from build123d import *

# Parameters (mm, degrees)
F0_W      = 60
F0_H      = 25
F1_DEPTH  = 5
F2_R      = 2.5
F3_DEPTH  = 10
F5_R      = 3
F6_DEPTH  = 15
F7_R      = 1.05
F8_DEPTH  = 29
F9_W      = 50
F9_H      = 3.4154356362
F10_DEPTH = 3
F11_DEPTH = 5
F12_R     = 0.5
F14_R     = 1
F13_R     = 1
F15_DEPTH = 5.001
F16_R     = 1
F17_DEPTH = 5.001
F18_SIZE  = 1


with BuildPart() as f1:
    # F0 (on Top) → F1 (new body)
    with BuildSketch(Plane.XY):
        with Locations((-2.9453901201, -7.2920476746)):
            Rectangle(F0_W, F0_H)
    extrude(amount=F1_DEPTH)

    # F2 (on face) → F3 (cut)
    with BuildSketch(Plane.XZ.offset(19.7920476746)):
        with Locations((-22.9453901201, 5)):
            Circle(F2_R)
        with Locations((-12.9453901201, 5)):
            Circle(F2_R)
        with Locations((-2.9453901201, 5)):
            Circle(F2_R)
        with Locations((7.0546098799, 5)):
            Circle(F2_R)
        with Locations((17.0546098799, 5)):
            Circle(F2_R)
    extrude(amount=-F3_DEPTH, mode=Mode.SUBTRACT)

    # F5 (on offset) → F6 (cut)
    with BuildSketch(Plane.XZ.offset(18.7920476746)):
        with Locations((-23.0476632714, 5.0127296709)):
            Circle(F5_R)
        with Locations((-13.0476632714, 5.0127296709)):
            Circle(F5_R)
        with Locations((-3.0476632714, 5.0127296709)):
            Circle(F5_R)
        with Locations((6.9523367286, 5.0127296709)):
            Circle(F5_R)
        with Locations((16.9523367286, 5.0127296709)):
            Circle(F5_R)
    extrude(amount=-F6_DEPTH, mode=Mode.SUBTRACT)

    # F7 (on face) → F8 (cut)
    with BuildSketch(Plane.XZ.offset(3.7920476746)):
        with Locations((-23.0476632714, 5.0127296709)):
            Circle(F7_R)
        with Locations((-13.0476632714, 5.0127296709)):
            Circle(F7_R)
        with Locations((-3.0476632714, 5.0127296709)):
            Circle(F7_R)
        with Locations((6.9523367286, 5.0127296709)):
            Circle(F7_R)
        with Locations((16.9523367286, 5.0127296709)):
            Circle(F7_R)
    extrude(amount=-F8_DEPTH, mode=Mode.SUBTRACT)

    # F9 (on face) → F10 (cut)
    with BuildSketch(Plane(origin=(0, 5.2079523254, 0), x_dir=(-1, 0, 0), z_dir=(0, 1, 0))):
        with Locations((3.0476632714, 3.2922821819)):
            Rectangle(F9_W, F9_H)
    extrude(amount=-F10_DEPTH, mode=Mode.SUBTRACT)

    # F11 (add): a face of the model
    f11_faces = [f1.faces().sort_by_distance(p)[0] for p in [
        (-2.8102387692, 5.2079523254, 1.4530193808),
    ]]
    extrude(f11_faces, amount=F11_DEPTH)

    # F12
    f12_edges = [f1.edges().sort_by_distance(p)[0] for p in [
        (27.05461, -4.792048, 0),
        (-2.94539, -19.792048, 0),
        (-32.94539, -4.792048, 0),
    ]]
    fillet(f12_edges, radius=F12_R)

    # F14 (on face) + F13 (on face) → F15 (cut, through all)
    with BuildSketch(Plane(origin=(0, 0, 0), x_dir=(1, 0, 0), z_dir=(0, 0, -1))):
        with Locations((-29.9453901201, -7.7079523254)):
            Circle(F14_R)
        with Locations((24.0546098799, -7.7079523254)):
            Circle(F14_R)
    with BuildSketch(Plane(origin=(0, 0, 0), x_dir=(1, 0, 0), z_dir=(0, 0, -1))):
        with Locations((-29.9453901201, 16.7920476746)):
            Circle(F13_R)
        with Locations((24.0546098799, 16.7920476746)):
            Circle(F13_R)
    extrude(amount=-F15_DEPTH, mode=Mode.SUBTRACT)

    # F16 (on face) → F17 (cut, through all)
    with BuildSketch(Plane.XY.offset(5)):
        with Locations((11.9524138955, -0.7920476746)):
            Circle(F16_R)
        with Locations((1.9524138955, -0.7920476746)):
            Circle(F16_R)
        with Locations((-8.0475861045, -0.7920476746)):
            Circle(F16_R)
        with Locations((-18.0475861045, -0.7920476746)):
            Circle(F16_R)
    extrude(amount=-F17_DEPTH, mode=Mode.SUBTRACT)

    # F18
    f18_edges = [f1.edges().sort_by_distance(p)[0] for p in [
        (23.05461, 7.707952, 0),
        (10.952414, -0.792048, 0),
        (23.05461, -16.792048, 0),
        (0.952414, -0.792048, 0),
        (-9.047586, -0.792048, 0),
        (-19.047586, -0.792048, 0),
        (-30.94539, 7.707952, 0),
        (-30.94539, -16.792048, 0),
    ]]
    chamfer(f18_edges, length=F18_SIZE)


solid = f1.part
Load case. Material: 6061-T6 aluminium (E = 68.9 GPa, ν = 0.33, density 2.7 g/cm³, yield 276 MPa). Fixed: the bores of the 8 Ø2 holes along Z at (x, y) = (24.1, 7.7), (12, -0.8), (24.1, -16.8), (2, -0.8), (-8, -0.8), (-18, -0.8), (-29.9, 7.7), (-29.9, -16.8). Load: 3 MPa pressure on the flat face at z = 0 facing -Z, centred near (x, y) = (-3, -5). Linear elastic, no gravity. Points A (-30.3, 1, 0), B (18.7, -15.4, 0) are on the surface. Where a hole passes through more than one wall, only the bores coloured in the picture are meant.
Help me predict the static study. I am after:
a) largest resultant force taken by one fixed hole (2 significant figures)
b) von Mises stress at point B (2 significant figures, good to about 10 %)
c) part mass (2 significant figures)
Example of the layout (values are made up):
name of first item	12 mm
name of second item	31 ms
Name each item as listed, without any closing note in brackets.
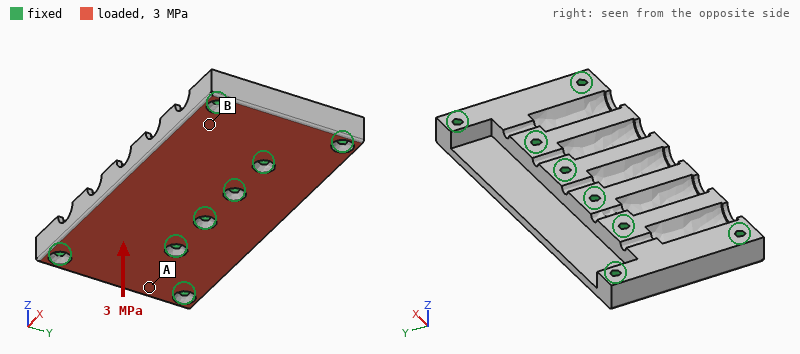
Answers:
largest resultant force taken by one fixed hole	860 N
von Mises stress at point B	53 MPa
part mass	17 g
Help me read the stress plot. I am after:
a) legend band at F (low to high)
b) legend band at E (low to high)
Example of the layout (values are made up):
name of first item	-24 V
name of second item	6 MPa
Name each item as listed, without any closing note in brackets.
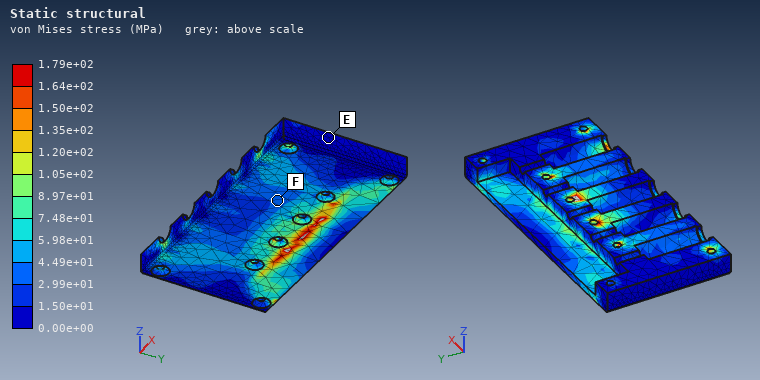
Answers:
legend band at F	2.99e+01 to 4.49e+01 MPa
legend band at E	0.00e+00 to 1.50e+01 MPa
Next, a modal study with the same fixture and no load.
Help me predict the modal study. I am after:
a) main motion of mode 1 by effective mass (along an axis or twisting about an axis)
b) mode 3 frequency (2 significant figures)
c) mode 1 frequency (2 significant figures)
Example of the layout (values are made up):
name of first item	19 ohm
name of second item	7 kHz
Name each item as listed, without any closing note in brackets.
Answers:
main motion of mode 1 by effective mass	along Z
mode 3 frequency	20 kHz
mode 1 frequency	13 kHz
